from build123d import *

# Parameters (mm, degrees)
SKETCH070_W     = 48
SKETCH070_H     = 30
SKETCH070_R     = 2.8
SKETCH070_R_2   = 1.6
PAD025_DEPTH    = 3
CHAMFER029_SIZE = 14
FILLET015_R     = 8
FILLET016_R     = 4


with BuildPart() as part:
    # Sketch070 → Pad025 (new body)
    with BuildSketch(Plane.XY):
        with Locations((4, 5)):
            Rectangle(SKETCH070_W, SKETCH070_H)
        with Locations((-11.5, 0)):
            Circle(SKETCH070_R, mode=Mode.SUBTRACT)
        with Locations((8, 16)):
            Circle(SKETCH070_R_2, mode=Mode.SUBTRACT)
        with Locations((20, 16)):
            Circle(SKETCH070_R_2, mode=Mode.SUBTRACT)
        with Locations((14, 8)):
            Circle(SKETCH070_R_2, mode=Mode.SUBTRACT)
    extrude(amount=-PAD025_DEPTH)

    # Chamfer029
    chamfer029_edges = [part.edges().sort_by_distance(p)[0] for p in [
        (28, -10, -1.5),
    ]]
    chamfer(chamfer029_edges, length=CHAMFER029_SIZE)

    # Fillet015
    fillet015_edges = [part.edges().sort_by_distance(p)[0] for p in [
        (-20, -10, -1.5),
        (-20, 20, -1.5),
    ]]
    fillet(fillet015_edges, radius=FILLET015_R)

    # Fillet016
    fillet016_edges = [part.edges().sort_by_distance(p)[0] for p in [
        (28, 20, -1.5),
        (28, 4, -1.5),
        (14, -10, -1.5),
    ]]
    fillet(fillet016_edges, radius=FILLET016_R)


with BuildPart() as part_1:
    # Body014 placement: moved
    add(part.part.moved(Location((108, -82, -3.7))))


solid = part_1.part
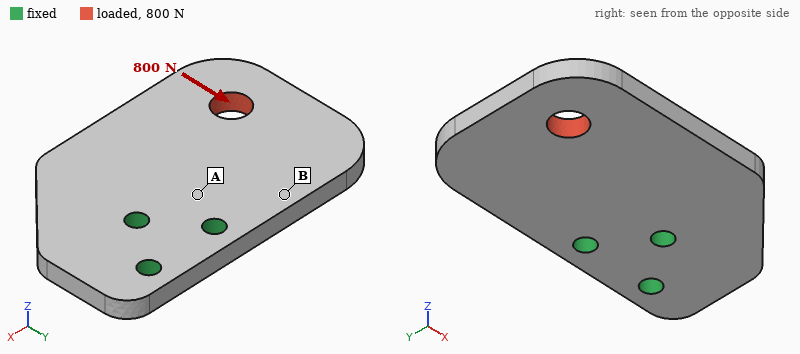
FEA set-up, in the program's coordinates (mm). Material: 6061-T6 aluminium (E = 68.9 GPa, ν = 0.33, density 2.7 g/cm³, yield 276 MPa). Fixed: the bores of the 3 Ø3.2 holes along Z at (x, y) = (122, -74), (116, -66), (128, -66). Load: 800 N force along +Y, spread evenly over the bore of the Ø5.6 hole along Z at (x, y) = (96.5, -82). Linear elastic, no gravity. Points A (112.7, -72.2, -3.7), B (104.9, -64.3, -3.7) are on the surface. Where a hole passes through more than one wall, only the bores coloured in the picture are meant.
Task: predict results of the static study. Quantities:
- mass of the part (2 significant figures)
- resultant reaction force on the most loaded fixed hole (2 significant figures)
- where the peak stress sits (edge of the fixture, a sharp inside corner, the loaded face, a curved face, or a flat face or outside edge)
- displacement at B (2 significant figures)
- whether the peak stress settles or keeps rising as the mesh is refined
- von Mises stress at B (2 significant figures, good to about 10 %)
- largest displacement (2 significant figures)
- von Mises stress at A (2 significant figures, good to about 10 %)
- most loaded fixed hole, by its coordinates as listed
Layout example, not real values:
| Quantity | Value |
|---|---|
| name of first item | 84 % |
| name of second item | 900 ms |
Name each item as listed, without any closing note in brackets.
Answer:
| Quantity | Value |
|---|---|
| mass of the part | 10 g |
| resultant reaction force on the most loaded fixed hole | 1.4 kN |
| where the peak stress sits | edge of the fixture |
| displacement at B | 17 µm |
| whether the peak stress settles or keeps rising as the mesh is refined | keeps rising |
| von Mises stress at B | 17 MPa |
| largest displacement | 41 µm |
| von Mises stress at A | 40 MPa |
| most loaded fixed hole, by its coordinates as listed | (116, -66) |
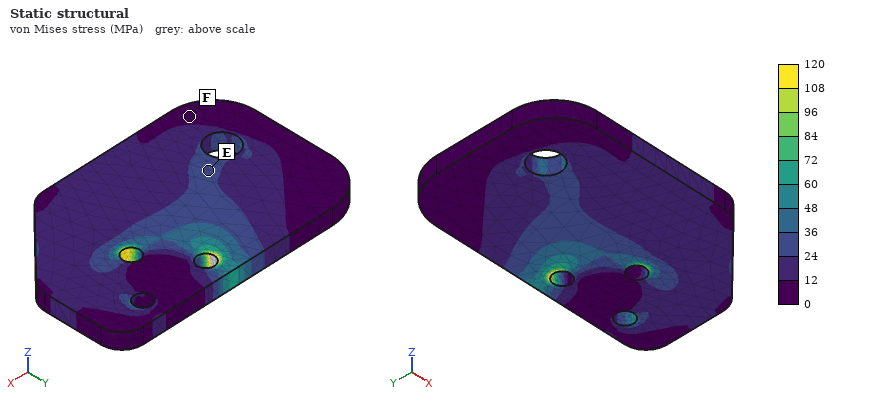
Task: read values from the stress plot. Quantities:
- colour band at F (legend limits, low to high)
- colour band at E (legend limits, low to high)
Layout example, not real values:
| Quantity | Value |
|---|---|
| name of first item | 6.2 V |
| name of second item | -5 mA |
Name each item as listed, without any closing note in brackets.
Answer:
| Quantity | Value |
|---|---|
| colour band at F | 0 to 12 MPa |
| colour band at E | 24 to 36 MPa |
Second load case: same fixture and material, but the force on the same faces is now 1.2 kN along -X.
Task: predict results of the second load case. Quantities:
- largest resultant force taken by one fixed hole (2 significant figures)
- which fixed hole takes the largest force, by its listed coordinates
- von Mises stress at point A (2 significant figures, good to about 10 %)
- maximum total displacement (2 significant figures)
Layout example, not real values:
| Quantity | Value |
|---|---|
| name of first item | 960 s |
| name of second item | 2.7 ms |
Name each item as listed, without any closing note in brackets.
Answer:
| Quantity | Value |
|---|---|
| largest resultant force taken by one fixed hole | 1.4 kN |
| which fixed hole takes the largest force, by its listed coordinates | (122, -74) |
| von Mises stress at point A | 28 MPa |
| maximum total displacement | 31 µm |
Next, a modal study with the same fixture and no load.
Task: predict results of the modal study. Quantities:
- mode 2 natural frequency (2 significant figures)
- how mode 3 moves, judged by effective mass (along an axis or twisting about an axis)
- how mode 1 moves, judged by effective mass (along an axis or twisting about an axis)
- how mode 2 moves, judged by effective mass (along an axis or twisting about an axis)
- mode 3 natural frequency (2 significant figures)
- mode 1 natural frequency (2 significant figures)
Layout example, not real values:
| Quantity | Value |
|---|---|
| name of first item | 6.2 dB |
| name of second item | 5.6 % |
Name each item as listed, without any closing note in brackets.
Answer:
| Quantity | Value |
|---|---|
| mode 2 natural frequency | 5600 Hz |
| how mode 3 moves, judged by effective mass | along Z |
| how mode 1 moves, judged by effective mass | along Z |
| how mode 2 moves, judged by effective mass | twisting about X |
| mode 3 natural frequency | 11 kHz |
| mode 1 natural frequency | 2500 Hz |
